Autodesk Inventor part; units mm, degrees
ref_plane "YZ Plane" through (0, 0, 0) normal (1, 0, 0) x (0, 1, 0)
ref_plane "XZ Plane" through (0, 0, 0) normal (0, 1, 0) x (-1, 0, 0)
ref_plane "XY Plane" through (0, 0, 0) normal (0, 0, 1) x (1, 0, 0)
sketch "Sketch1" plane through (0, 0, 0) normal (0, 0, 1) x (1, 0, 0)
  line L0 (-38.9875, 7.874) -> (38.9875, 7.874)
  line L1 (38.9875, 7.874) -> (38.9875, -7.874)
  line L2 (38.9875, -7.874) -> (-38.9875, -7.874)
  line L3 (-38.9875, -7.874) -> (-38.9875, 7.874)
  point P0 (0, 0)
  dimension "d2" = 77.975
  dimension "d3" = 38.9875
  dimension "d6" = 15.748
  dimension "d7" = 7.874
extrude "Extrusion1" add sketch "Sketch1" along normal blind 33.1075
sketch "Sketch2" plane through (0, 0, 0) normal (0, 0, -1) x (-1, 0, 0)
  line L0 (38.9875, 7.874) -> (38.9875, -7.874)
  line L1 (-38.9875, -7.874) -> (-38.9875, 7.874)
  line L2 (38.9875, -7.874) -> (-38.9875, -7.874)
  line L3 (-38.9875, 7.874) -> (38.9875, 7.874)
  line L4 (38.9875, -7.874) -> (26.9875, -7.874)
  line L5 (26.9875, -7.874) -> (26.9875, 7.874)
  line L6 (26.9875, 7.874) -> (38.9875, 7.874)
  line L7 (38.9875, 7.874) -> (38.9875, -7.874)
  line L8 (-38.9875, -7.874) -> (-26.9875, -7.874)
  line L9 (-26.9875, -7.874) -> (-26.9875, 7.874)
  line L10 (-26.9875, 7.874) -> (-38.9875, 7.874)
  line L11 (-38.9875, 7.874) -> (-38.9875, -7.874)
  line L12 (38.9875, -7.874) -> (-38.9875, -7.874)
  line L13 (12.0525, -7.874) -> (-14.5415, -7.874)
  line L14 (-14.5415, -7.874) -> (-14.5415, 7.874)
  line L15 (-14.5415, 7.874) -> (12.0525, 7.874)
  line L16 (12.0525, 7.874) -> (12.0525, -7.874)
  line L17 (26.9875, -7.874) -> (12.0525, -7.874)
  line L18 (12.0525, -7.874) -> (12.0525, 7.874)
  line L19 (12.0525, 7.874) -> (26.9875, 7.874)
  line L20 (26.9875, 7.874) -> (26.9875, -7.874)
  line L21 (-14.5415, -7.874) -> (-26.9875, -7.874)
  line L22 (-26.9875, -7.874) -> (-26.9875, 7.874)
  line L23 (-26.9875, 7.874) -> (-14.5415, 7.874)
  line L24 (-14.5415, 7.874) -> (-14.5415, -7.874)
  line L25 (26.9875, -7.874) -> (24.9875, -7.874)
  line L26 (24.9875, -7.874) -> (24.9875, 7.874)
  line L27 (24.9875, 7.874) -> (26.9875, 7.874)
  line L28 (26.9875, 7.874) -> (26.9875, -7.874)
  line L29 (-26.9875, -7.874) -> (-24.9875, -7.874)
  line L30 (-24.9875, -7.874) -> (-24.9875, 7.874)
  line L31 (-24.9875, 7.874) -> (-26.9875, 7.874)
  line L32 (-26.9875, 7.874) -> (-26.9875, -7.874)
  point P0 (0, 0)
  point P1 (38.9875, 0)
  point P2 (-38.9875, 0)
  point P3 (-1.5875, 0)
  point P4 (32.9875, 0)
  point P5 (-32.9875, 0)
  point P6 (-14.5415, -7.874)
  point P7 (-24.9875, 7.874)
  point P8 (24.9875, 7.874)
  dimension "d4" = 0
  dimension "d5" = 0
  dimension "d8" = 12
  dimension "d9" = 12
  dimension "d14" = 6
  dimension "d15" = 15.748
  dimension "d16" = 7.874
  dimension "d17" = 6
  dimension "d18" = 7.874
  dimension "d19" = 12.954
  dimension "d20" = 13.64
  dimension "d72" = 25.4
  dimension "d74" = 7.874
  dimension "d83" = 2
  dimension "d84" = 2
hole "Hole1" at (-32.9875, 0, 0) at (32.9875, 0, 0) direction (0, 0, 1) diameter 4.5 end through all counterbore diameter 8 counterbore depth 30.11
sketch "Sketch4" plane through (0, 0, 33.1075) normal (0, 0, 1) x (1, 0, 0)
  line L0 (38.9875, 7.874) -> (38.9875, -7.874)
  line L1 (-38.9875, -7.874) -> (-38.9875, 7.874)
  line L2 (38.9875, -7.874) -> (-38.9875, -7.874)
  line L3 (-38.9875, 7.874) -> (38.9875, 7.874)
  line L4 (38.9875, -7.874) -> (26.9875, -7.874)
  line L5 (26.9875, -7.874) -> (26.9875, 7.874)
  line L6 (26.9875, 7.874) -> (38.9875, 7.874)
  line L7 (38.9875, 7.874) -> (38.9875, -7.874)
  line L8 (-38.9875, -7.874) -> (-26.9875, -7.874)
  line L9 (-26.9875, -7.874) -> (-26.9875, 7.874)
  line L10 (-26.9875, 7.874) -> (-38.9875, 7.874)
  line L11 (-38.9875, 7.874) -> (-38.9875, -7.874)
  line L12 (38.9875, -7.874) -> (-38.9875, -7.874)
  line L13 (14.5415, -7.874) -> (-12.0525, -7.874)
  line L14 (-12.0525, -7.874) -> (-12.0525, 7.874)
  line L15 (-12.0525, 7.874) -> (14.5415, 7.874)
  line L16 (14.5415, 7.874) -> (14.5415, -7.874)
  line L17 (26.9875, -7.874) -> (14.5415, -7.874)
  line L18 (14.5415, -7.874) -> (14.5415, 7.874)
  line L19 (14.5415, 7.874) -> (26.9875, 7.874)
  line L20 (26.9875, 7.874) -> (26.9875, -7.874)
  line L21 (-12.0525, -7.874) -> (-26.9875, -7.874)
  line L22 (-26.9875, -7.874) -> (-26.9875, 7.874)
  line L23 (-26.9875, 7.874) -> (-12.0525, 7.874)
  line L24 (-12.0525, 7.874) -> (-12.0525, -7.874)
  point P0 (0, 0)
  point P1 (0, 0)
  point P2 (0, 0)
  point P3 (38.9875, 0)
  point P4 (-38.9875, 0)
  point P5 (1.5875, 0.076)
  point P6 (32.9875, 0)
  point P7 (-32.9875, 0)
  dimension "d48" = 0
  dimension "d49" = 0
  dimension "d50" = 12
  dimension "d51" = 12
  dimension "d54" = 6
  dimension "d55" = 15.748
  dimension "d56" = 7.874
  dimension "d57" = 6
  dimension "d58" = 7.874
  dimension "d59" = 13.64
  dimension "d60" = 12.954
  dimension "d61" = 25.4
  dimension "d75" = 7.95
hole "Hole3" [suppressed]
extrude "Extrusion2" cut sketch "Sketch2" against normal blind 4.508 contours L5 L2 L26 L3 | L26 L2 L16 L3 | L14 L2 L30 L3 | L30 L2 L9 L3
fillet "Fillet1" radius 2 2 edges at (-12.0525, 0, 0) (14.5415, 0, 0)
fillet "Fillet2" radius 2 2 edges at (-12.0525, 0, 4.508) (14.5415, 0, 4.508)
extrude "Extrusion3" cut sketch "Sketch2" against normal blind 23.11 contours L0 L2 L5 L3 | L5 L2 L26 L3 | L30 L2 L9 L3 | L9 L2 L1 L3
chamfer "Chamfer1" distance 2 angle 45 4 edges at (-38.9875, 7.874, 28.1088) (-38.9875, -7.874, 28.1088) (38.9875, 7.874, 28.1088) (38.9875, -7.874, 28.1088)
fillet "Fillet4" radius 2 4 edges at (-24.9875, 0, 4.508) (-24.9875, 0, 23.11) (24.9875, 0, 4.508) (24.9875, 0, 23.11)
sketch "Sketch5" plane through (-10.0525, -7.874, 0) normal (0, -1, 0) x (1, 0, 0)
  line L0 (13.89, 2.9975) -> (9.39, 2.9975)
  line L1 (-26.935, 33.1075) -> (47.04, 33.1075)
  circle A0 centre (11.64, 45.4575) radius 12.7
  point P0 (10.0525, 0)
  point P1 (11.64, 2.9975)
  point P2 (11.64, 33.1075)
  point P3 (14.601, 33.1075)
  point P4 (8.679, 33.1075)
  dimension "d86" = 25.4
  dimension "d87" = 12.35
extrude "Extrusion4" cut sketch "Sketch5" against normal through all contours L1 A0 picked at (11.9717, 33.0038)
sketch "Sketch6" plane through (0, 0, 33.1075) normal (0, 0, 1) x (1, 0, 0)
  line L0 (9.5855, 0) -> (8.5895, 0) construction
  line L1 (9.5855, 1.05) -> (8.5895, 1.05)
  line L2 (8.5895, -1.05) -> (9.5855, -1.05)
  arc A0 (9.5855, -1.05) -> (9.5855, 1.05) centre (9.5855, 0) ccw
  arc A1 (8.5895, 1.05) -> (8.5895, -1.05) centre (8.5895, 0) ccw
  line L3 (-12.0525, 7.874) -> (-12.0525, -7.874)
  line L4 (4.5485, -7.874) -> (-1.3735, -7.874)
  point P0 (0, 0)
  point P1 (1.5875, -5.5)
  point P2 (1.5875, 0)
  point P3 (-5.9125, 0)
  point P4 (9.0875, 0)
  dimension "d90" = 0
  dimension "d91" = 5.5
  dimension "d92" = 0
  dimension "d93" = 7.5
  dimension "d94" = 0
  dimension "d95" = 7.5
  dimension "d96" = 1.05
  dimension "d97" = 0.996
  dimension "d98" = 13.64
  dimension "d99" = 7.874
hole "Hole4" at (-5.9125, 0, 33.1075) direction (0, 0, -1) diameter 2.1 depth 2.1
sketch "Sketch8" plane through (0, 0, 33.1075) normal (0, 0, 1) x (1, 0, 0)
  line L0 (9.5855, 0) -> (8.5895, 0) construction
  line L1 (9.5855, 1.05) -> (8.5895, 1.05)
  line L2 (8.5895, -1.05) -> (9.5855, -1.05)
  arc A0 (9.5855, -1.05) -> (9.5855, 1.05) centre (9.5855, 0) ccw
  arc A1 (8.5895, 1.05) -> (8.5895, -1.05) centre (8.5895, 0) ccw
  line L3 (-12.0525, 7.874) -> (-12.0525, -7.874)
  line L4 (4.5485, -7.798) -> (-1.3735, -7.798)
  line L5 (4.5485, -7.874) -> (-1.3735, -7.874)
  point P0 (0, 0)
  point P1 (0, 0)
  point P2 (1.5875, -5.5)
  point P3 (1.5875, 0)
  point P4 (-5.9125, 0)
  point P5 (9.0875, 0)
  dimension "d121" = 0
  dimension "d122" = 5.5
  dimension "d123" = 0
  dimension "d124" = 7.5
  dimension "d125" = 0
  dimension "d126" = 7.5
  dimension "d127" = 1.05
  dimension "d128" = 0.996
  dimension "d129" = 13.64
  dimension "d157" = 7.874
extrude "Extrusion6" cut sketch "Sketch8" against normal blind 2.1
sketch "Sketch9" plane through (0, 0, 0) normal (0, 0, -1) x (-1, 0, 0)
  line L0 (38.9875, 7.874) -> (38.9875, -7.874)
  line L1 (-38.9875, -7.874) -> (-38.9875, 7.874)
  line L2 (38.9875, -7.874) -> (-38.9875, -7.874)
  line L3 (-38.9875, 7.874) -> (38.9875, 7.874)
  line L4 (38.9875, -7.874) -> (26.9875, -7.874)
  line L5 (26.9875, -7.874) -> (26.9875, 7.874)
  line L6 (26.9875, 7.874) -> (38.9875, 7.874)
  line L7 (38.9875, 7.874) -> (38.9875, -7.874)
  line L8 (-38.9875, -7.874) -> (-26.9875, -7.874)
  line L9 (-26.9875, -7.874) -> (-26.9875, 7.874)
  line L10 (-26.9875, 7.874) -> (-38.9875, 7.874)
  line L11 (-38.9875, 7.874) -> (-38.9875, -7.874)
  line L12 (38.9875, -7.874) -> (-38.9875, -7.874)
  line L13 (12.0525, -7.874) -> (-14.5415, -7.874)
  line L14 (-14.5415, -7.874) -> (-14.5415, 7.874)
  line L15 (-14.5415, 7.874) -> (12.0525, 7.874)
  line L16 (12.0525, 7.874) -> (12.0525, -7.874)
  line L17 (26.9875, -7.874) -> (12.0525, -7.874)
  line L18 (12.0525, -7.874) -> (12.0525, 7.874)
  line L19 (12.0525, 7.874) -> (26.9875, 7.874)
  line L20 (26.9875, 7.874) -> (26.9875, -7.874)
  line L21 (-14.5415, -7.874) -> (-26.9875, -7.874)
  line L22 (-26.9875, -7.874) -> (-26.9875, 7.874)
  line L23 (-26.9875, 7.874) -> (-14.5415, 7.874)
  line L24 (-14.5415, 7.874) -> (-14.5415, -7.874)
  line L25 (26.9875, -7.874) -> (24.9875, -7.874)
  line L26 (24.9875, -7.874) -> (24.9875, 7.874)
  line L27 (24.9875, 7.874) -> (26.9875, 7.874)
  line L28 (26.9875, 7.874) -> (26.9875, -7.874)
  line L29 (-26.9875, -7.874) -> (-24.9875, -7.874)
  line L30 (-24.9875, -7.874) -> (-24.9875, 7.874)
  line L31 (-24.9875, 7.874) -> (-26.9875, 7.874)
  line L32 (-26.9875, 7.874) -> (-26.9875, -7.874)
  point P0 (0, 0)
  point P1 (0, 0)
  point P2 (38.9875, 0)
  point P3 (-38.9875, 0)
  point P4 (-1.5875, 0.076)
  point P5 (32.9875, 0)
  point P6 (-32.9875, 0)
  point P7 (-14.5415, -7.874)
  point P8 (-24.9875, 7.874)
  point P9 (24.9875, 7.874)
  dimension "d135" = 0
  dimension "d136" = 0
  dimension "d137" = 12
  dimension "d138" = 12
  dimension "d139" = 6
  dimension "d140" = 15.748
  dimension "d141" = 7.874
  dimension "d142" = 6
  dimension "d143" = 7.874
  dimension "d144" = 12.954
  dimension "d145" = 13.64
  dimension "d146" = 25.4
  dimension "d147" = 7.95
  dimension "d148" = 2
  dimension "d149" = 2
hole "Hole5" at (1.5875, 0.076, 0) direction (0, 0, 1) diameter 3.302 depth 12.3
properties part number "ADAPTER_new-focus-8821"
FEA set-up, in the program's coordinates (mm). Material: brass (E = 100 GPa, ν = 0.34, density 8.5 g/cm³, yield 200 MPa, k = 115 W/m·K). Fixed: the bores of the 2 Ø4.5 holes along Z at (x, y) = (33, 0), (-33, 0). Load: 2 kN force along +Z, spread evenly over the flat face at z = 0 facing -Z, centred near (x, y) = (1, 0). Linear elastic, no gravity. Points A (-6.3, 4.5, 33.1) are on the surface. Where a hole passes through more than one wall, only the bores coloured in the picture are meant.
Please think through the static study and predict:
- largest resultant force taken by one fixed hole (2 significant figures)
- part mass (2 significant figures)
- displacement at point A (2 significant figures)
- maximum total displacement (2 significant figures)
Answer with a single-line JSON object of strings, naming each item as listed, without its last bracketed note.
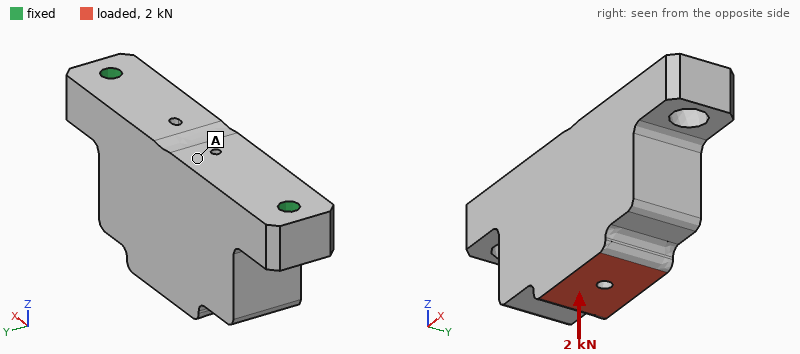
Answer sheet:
{"largest resultant force taken by one fixed hole": "1.3 kN", "part mass": "240 g", "displacement at point A": "7.0 µm", "maximum total displacement": "7.9 µm"}
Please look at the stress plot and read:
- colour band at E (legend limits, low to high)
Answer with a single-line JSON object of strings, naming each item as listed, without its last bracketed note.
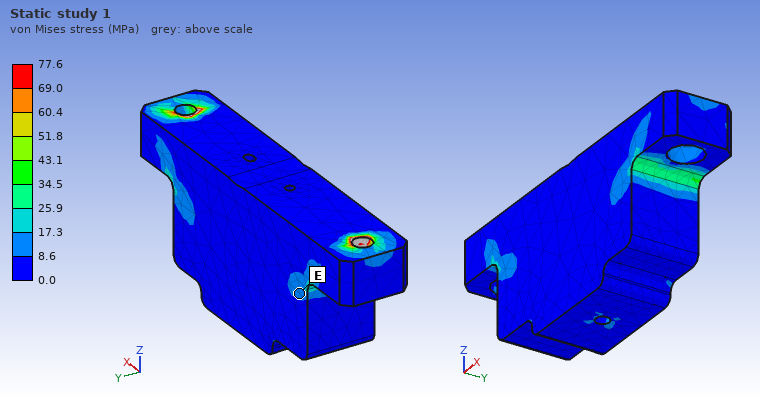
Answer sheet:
{"colour band at E": "8.6 to 17.3 MPa"}
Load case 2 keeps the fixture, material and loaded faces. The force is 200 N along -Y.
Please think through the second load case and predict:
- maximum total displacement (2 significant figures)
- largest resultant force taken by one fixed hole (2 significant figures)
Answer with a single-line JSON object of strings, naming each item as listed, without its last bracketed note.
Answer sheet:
{"maximum total displacement": "33 µm", "largest resultant force taken by one fixed hole": "100 N"}
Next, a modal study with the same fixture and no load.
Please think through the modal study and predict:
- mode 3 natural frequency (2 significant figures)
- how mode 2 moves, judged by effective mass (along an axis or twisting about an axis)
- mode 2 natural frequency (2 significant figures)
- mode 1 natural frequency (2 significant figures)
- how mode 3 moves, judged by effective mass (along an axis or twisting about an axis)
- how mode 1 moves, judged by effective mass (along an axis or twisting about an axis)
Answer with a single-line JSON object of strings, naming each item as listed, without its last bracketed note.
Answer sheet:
{"mode 3 natural frequency": "7500 Hz", "how mode 2 moves, judged by effective mass": "along Z", "mode 2 natural frequency": "6000 Hz", "mode 1 natural frequency": "1600 Hz", "how mode 3 moves, judged by effective mass": "along Y", "how mode 1 moves, judged by effective mass": "along Y"}
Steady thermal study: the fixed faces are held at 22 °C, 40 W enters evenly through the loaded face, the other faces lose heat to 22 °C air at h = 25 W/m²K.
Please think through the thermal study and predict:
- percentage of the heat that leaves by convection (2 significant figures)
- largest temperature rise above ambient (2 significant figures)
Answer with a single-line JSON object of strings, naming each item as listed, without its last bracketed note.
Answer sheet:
{"percentage of the heat that leaves by convection": "9.2 %", "largest temperature rise above ambient": "39 K"}
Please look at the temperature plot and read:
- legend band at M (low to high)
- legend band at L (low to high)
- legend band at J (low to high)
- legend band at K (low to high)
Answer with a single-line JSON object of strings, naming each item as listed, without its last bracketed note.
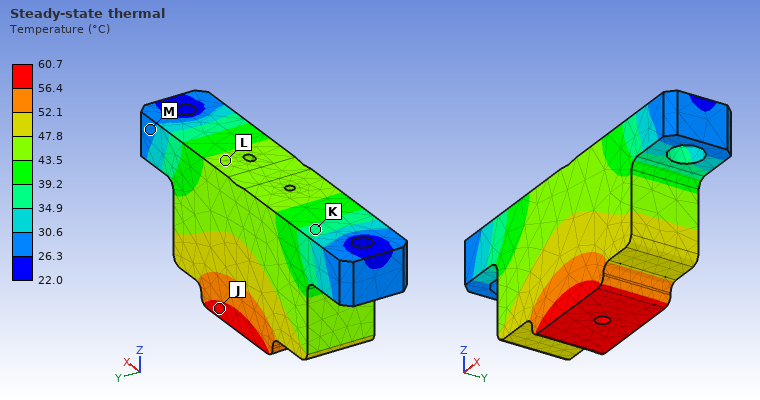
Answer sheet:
{"legend band at M": "26.3 to 30.6 °C", "legend band at L": "43.5 to 47.8 °C", "legend band at J": "56.4 to 60.7 °C", "legend band at K": "34.9 to 39.2 °C"}
